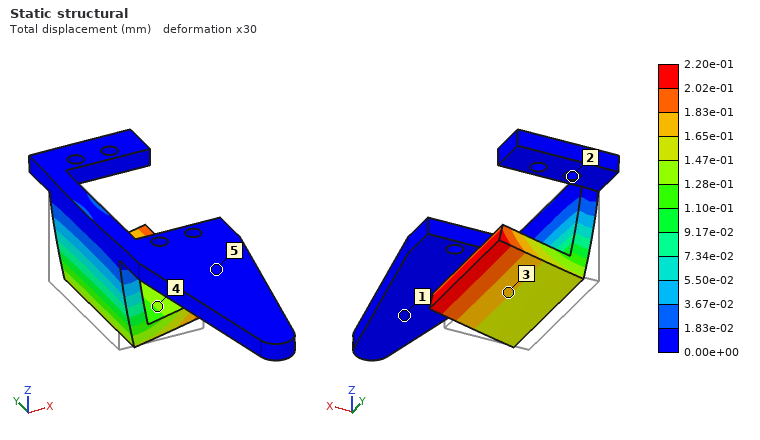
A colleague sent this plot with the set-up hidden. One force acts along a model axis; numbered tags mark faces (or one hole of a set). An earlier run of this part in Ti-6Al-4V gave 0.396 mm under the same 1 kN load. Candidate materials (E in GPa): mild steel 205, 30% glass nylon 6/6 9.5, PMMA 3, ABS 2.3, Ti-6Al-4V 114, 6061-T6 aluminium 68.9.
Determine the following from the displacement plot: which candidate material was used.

mild steel
